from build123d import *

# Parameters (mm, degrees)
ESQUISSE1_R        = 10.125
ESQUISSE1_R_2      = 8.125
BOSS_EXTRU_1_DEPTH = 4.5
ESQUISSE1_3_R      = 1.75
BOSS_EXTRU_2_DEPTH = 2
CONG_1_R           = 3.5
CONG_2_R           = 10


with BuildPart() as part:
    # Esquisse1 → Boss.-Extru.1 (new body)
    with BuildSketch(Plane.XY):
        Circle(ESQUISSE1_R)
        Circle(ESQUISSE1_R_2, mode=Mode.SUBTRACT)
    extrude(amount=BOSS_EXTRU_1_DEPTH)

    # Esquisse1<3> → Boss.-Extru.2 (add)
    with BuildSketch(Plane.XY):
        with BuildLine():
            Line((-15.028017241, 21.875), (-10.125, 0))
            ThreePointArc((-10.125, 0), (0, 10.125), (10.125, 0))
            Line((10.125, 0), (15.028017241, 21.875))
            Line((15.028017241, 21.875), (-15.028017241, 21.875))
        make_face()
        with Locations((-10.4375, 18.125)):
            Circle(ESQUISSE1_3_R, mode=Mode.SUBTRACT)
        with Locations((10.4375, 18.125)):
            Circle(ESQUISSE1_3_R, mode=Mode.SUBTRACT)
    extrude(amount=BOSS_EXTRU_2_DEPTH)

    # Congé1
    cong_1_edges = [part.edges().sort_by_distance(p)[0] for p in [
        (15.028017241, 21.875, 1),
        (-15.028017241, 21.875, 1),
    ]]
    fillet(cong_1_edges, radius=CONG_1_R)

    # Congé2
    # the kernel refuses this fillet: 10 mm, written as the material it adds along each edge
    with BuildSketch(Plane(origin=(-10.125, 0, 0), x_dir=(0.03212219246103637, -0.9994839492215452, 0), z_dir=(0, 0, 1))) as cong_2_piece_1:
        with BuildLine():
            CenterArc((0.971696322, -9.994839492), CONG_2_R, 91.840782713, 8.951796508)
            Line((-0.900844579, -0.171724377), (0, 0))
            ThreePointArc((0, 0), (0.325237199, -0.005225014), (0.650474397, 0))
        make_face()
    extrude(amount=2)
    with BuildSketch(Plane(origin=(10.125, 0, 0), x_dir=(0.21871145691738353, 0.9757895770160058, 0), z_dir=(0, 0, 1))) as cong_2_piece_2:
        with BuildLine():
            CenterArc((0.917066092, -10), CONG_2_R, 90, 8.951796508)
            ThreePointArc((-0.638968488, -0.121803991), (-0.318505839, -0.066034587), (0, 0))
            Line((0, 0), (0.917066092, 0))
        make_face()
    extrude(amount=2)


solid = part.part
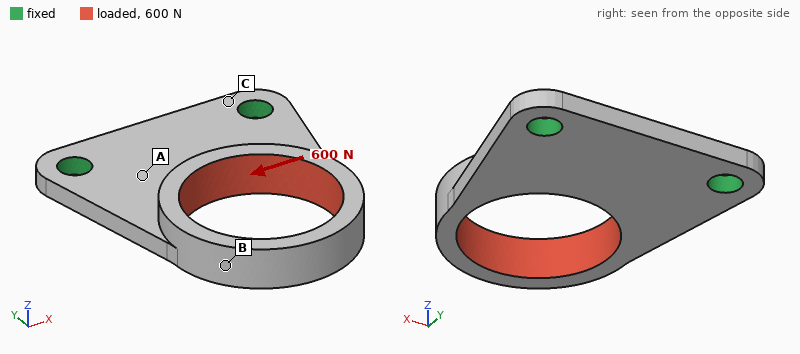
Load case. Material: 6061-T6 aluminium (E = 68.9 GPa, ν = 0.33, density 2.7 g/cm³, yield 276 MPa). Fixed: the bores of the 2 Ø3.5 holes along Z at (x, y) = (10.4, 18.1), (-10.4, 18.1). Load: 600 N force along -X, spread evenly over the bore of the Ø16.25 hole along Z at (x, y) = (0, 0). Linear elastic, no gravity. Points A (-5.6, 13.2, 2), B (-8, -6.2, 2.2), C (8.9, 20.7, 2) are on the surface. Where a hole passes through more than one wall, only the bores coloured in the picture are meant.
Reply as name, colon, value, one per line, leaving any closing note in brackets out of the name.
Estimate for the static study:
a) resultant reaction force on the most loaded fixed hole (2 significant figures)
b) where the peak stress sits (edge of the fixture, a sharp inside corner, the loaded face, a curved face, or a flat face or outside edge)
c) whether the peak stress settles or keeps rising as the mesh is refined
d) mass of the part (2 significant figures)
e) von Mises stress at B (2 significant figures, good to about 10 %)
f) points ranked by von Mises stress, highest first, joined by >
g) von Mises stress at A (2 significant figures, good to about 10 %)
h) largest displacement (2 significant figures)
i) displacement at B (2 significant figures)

resultant reaction force on the most loaded fixed hole: 570 N
where the peak stress sits: a sharp inside corner
whether the peak stress settles or keeps rising as the mesh is refined: keeps rising
mass of the part: 3.3 g
von Mises stress at B: 90 MPa
points ranked by von Mises stress, highest first, joined by >: B > A > C
von Mises stress at A: 37 MPa
largest displacement: 0.11 mm
displacement at B: 0.10 mm
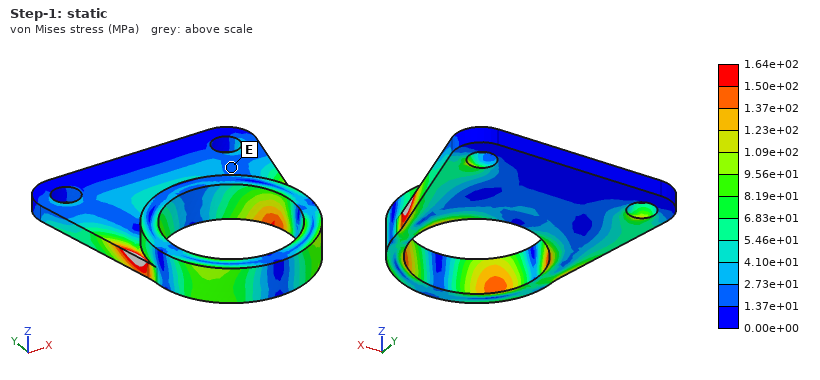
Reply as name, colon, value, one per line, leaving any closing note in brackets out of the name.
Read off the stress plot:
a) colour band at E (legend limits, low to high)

colour band at E: 1.37e+01 to 2.73e+01 MPa
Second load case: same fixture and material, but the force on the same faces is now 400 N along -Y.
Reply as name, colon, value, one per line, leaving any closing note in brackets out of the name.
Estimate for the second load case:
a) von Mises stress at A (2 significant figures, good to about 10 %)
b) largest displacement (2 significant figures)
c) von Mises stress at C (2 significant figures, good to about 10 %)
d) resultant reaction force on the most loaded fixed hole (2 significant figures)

von Mises stress at A: 31 MPa
largest displacement: 0.13 mm
von Mises stress at C: 12 MPa
resultant reaction force on the most loaded fixed hole: 200 N
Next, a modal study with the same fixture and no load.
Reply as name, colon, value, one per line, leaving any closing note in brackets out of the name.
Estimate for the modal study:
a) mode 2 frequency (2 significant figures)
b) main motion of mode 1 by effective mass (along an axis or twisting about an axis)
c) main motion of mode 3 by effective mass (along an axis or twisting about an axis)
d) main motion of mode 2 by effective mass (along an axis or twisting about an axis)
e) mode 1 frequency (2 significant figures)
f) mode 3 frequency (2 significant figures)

mode 2 frequency: 8400 Hz
main motion of mode 1 by effective mass: along Z
main motion of mode 3 by effective mass: along X
main motion of mode 2 by effective mass: twisting about Y
mode 1 frequency: 2800 Hz
mode 3 frequency: 11 kHz
